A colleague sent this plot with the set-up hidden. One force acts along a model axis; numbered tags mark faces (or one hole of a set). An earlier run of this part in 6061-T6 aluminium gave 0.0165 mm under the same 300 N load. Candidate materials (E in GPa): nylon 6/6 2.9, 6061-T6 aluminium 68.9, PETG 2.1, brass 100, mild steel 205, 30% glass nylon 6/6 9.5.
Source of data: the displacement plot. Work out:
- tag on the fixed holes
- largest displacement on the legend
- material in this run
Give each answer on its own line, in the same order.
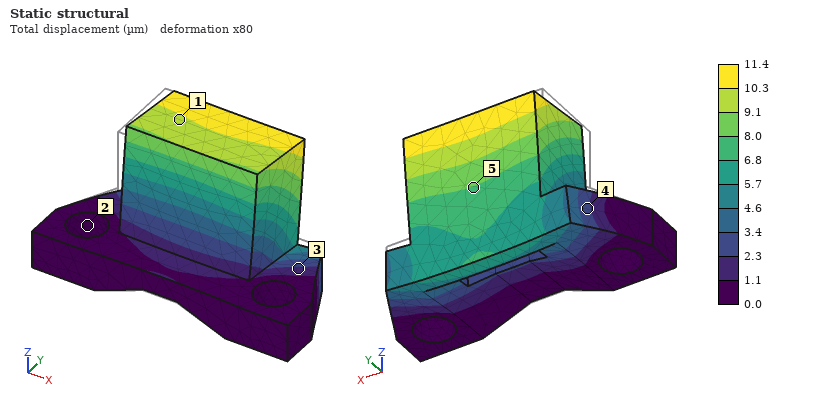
2
11.4 µm
brass
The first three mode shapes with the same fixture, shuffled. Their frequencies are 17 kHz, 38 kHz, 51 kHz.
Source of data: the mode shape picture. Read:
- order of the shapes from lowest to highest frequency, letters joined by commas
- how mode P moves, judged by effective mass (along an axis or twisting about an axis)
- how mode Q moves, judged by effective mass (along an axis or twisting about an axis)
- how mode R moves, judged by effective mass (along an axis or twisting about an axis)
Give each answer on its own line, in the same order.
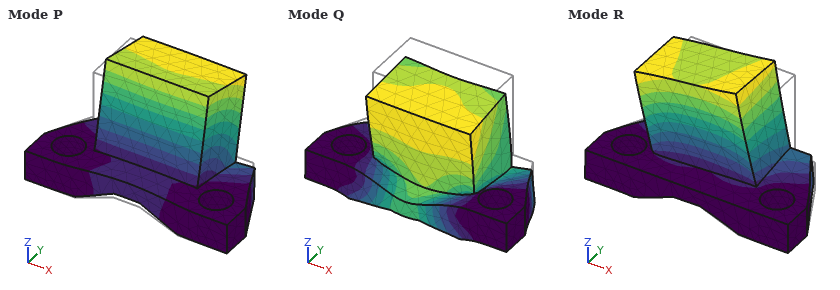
P, R, Q
along Y
along Z
along X
